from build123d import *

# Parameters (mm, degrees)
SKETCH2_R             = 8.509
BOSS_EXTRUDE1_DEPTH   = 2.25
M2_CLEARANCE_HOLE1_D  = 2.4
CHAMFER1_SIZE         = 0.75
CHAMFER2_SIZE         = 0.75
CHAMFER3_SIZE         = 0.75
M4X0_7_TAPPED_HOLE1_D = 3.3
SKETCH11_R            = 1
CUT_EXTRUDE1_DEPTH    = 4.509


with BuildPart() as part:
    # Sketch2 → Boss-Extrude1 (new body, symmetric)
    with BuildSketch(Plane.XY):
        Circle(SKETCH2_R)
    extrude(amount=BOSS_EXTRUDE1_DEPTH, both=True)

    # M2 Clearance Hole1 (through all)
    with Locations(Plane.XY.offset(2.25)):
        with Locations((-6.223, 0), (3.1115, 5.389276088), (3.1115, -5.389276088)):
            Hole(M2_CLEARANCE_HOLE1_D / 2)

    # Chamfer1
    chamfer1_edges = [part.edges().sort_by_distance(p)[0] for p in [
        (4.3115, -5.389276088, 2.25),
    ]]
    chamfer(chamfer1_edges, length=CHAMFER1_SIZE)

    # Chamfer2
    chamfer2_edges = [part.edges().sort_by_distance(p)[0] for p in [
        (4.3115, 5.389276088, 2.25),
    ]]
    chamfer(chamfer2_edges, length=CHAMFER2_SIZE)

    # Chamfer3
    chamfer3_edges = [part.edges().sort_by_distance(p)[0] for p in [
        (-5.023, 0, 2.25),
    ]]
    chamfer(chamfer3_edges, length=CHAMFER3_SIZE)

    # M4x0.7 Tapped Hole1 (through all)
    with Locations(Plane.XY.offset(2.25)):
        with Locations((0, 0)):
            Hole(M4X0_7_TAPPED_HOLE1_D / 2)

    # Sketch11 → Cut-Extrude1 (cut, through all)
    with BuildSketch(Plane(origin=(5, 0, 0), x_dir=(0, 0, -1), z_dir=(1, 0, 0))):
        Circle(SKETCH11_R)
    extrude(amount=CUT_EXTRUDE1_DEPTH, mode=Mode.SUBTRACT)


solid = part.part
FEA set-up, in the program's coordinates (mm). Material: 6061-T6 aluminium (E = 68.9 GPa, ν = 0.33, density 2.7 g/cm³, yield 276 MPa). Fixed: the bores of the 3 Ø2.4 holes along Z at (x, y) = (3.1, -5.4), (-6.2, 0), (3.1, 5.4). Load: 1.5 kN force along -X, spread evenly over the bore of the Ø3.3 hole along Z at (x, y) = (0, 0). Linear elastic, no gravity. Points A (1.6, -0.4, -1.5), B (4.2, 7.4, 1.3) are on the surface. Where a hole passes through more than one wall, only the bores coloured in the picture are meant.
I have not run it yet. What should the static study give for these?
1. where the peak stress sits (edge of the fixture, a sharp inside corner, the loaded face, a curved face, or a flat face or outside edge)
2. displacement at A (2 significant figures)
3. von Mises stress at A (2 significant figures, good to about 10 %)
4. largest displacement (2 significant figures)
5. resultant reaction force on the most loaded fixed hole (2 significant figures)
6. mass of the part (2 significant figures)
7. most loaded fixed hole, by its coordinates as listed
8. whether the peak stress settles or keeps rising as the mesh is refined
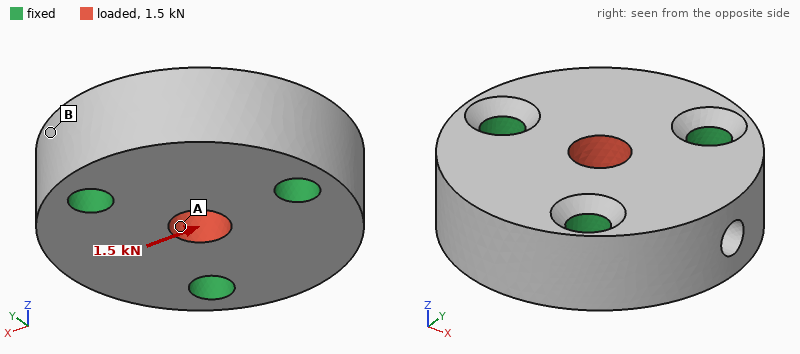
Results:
edge of the fixture
2.8 µm
30 MPa
3.1 µm
550 N
2.4 g
(-6.2, 0)
keeps rising
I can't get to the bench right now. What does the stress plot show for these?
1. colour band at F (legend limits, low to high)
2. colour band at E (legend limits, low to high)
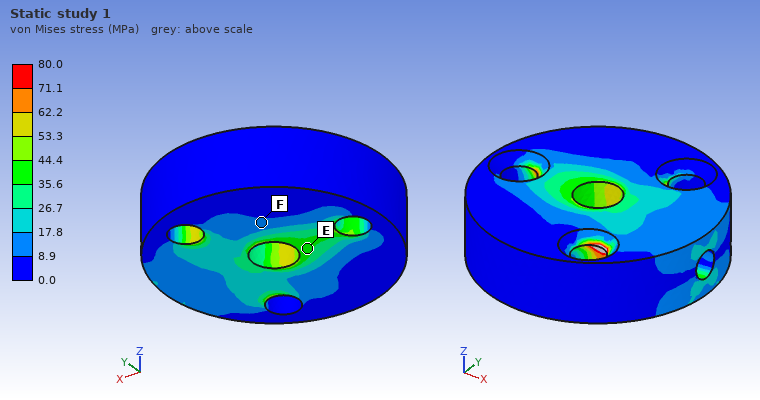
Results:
8.9 to 17.8 MPa
35.6 to 44.4 MPa
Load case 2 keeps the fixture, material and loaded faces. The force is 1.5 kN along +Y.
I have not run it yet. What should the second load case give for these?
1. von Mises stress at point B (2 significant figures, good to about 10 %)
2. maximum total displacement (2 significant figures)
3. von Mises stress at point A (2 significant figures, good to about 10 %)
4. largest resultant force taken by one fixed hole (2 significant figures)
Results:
6.1 MPa
2.8 µm
54 MPa
520 N
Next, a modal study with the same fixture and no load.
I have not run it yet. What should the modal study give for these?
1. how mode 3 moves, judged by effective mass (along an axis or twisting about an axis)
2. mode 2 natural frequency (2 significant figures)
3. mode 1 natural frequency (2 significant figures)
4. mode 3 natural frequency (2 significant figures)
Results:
along Z
83 kHz
81 kHz
91 kHz
